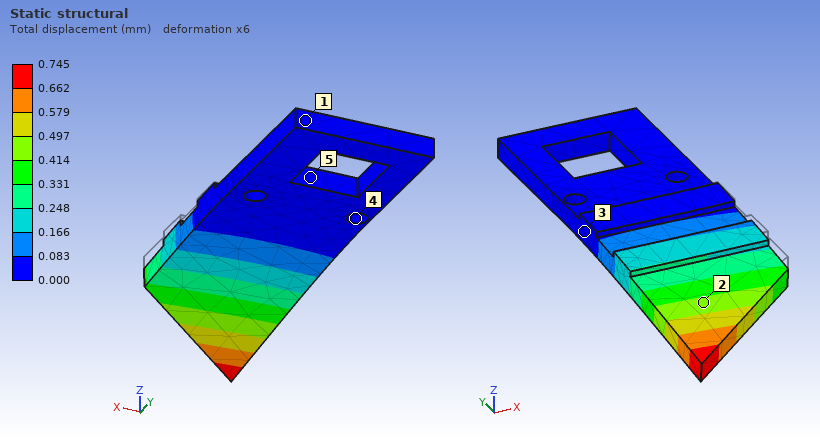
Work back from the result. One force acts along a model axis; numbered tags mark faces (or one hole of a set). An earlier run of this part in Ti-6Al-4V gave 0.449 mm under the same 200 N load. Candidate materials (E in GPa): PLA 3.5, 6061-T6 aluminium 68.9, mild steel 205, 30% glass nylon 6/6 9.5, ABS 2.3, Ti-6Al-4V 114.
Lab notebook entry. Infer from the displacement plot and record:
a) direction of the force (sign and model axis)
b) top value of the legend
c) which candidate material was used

-Z
0.745 mm
6061-T6 aluminium
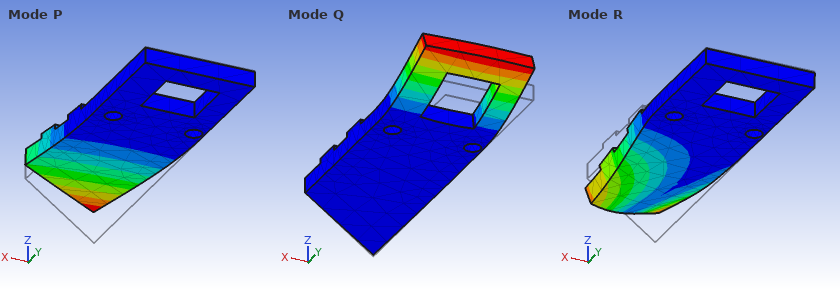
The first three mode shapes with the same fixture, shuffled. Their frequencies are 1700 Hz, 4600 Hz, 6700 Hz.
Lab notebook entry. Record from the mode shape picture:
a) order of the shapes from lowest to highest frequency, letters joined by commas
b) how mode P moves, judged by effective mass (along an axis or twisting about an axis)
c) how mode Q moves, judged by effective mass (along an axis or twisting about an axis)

P, Q, R
along Z
along Z
